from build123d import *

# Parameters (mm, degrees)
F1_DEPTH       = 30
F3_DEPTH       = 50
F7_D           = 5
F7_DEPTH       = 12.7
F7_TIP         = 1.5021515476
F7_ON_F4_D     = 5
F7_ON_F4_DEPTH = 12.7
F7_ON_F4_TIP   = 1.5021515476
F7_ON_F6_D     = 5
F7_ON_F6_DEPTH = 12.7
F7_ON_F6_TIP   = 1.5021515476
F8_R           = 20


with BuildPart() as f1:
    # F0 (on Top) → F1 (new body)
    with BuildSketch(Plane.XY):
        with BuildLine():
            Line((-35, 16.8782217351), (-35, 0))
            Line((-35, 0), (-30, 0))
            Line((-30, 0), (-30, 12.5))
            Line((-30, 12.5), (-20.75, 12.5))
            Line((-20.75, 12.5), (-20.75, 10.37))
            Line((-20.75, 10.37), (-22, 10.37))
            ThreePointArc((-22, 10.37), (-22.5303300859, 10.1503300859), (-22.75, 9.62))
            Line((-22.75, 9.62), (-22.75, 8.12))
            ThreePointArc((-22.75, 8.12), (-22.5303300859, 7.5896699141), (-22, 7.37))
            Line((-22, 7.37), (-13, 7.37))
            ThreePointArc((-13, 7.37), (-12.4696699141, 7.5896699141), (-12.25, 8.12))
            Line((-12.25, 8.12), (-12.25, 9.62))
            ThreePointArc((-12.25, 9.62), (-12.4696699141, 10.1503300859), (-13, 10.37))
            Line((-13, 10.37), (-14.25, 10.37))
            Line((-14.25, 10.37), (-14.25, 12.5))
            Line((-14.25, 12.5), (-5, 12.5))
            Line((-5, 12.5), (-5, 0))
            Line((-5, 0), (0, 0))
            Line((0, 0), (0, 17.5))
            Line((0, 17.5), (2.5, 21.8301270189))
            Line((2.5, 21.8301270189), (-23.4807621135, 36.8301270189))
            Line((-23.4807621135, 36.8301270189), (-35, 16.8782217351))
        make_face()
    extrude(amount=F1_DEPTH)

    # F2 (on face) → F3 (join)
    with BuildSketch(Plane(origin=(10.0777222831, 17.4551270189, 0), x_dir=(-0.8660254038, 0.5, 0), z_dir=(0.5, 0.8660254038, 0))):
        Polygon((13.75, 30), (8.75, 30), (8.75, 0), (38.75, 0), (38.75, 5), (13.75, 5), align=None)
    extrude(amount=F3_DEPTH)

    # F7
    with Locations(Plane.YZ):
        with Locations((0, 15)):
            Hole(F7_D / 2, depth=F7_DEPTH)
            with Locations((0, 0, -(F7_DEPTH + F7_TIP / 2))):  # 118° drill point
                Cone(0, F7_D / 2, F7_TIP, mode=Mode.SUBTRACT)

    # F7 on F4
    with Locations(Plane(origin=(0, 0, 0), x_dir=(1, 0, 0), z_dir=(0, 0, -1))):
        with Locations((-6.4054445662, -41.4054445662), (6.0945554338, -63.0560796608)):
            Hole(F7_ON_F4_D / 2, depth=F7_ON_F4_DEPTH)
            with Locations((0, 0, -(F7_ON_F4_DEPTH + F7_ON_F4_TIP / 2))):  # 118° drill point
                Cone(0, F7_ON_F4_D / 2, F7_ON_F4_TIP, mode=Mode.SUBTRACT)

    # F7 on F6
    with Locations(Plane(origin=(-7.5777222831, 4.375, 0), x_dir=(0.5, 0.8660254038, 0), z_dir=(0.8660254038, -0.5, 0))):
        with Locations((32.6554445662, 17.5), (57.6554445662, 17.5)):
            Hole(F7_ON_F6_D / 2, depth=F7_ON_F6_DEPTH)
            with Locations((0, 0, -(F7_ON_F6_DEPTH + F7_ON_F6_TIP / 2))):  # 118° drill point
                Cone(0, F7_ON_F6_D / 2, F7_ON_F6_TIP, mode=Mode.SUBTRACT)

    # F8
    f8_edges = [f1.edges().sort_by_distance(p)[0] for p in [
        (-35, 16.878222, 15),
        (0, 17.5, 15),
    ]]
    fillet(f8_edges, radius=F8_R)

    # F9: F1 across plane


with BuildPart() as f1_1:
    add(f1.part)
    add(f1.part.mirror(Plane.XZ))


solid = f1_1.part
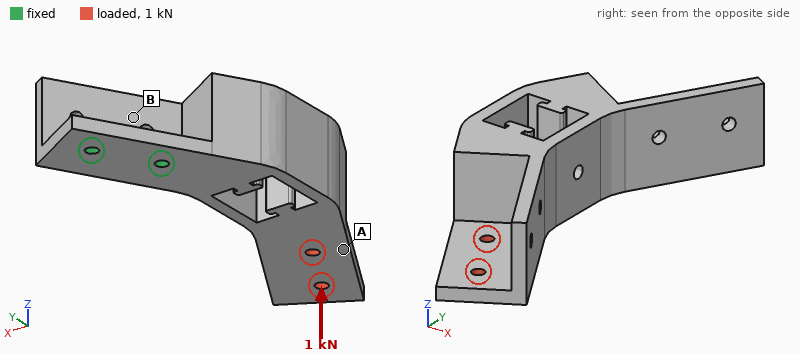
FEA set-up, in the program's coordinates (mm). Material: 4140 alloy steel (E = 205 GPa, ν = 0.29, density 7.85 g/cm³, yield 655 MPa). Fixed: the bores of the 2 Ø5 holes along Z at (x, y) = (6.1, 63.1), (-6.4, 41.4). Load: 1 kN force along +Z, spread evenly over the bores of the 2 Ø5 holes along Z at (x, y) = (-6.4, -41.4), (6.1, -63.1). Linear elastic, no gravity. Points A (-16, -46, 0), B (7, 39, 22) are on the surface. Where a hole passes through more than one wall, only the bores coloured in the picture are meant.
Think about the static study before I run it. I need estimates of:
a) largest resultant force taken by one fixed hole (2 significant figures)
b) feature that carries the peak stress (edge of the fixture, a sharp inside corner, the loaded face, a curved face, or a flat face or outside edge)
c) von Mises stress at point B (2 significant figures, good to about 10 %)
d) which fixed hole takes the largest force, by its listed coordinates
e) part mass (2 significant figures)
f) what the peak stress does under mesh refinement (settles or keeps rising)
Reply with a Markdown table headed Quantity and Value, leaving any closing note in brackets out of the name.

| Quantity | Value |
|---|---|
| largest resultant force taken by one fixed hole | 3.2 kN |
| feature that carries the peak stress | edge of the fixture |
| von Mises stress at point B | 72 MPa |
| which fixed hole takes the largest force, by its listed coordinates | (-6.4, 41.4) |
| part mass | 560 g |
| what the peak stress does under mesh refinement | keeps rising |
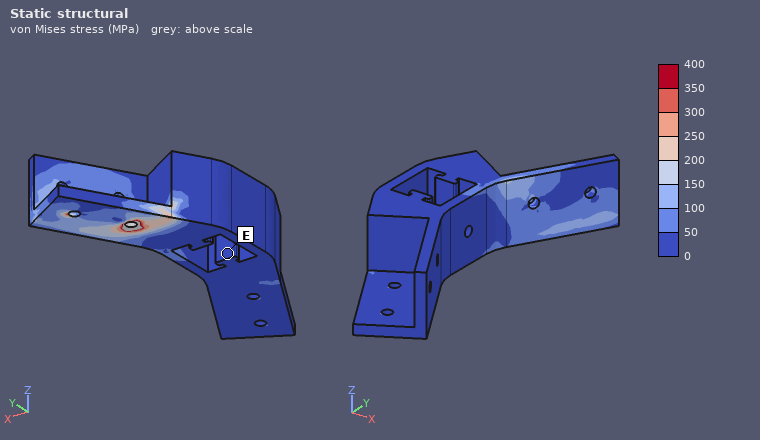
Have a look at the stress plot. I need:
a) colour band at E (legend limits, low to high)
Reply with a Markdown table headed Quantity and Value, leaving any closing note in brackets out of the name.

| Quantity | Value |
|---|---|
| colour band at E | 0 to 50 MPa |
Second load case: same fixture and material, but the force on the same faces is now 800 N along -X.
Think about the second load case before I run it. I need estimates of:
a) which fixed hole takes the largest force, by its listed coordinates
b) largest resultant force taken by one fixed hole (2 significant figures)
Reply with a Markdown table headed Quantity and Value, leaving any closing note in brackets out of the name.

| Quantity | Value |
|---|---|
| which fixed hole takes the largest force, by its listed coordinates | (-6.4, 41.4) |
| largest resultant force taken by one fixed hole | 3.1 kN |
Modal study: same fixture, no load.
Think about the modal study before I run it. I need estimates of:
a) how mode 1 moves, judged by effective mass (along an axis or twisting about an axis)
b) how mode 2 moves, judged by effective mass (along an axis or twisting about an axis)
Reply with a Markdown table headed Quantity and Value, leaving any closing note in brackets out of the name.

| Quantity | Value |
|---|---|
| how mode 1 moves, judged by effective mass | along Z |
| how mode 2 moves, judged by effective mass | along X |
